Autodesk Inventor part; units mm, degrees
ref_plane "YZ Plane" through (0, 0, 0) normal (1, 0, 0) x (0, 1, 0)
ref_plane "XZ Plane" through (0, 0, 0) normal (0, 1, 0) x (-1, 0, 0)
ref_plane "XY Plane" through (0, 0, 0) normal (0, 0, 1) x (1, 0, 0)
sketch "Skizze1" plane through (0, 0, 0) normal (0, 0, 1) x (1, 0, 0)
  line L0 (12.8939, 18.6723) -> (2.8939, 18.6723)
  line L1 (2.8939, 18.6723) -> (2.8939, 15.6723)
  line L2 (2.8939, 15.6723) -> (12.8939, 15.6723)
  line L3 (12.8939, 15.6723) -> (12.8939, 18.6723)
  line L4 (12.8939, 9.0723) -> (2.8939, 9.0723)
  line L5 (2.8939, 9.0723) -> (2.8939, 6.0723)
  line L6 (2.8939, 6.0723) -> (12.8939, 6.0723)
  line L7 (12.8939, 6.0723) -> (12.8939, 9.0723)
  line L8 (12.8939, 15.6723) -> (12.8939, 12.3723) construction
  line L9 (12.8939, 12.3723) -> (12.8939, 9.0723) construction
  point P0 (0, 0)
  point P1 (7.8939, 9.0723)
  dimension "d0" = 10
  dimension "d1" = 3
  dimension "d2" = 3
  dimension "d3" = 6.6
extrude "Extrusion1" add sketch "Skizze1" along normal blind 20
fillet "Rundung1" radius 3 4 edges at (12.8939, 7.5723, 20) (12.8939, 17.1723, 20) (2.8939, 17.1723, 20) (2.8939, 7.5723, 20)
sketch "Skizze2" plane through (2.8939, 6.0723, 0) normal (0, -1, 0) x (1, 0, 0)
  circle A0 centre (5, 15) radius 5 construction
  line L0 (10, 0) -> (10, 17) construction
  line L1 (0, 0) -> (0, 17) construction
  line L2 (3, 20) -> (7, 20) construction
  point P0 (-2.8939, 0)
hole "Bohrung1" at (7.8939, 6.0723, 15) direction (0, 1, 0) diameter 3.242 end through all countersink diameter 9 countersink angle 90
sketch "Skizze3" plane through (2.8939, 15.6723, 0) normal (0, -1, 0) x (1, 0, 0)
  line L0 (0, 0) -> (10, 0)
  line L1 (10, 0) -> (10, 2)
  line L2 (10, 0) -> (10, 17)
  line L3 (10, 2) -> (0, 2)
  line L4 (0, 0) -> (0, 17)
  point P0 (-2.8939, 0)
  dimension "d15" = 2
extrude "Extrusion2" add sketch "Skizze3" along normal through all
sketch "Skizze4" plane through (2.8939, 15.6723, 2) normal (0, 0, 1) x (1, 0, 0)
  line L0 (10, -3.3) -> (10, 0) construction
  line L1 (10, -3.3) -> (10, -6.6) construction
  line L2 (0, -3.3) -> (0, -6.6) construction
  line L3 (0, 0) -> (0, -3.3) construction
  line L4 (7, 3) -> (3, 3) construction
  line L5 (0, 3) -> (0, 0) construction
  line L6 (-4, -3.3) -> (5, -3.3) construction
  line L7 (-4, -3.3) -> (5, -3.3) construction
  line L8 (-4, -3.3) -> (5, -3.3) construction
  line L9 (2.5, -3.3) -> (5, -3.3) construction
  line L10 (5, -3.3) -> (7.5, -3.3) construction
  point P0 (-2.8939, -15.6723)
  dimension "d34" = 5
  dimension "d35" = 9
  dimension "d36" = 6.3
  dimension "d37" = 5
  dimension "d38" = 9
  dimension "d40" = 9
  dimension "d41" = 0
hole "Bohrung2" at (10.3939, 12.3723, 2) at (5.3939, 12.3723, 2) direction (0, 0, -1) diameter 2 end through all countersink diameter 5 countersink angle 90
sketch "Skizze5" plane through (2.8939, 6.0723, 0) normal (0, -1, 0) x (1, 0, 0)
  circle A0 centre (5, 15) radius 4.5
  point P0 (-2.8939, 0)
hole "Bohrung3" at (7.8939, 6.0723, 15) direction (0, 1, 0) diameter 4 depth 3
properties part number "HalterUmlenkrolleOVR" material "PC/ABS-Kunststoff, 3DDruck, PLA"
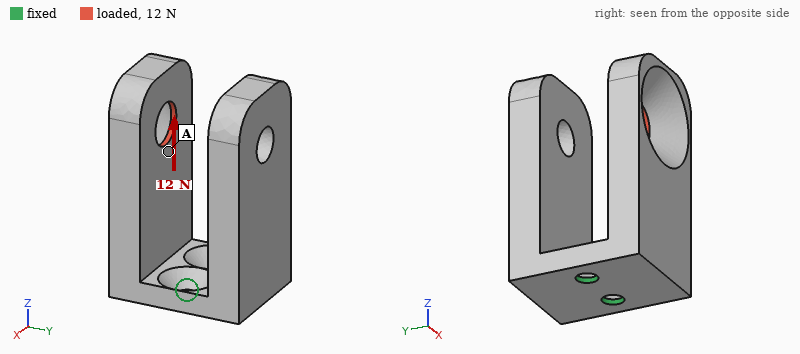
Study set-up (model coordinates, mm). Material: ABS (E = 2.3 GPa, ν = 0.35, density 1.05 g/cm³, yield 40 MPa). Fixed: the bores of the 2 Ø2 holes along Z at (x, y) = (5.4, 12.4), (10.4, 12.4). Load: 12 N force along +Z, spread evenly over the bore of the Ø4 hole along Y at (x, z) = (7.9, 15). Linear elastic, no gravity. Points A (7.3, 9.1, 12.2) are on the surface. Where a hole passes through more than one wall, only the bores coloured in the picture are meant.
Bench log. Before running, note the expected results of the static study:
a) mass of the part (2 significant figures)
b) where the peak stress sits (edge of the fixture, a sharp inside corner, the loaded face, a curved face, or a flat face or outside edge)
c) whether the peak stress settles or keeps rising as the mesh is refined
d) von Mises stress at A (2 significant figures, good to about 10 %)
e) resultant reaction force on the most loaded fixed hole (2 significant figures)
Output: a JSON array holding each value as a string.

["1.2 g", "edge of the fixture", "keeps rising", "2.0 MPa", "6.0 N"]
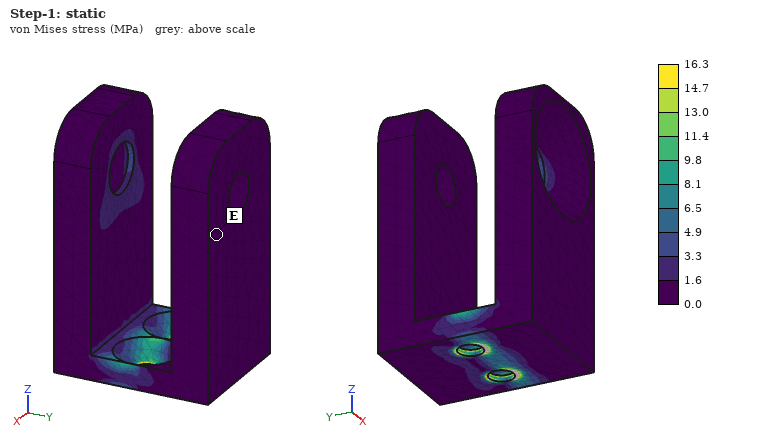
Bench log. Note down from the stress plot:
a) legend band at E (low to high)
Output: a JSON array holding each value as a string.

["0.0 to 1.6 MPa"]
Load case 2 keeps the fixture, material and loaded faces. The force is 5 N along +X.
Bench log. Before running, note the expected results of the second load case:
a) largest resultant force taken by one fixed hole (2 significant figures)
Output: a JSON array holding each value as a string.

["14 N"]
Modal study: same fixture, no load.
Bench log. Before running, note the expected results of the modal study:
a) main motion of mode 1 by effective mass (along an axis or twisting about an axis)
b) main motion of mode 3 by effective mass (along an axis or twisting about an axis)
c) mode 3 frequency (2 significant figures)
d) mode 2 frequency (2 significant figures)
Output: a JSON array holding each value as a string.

["along Y", "along X", "1600 Hz", "910 Hz"]
